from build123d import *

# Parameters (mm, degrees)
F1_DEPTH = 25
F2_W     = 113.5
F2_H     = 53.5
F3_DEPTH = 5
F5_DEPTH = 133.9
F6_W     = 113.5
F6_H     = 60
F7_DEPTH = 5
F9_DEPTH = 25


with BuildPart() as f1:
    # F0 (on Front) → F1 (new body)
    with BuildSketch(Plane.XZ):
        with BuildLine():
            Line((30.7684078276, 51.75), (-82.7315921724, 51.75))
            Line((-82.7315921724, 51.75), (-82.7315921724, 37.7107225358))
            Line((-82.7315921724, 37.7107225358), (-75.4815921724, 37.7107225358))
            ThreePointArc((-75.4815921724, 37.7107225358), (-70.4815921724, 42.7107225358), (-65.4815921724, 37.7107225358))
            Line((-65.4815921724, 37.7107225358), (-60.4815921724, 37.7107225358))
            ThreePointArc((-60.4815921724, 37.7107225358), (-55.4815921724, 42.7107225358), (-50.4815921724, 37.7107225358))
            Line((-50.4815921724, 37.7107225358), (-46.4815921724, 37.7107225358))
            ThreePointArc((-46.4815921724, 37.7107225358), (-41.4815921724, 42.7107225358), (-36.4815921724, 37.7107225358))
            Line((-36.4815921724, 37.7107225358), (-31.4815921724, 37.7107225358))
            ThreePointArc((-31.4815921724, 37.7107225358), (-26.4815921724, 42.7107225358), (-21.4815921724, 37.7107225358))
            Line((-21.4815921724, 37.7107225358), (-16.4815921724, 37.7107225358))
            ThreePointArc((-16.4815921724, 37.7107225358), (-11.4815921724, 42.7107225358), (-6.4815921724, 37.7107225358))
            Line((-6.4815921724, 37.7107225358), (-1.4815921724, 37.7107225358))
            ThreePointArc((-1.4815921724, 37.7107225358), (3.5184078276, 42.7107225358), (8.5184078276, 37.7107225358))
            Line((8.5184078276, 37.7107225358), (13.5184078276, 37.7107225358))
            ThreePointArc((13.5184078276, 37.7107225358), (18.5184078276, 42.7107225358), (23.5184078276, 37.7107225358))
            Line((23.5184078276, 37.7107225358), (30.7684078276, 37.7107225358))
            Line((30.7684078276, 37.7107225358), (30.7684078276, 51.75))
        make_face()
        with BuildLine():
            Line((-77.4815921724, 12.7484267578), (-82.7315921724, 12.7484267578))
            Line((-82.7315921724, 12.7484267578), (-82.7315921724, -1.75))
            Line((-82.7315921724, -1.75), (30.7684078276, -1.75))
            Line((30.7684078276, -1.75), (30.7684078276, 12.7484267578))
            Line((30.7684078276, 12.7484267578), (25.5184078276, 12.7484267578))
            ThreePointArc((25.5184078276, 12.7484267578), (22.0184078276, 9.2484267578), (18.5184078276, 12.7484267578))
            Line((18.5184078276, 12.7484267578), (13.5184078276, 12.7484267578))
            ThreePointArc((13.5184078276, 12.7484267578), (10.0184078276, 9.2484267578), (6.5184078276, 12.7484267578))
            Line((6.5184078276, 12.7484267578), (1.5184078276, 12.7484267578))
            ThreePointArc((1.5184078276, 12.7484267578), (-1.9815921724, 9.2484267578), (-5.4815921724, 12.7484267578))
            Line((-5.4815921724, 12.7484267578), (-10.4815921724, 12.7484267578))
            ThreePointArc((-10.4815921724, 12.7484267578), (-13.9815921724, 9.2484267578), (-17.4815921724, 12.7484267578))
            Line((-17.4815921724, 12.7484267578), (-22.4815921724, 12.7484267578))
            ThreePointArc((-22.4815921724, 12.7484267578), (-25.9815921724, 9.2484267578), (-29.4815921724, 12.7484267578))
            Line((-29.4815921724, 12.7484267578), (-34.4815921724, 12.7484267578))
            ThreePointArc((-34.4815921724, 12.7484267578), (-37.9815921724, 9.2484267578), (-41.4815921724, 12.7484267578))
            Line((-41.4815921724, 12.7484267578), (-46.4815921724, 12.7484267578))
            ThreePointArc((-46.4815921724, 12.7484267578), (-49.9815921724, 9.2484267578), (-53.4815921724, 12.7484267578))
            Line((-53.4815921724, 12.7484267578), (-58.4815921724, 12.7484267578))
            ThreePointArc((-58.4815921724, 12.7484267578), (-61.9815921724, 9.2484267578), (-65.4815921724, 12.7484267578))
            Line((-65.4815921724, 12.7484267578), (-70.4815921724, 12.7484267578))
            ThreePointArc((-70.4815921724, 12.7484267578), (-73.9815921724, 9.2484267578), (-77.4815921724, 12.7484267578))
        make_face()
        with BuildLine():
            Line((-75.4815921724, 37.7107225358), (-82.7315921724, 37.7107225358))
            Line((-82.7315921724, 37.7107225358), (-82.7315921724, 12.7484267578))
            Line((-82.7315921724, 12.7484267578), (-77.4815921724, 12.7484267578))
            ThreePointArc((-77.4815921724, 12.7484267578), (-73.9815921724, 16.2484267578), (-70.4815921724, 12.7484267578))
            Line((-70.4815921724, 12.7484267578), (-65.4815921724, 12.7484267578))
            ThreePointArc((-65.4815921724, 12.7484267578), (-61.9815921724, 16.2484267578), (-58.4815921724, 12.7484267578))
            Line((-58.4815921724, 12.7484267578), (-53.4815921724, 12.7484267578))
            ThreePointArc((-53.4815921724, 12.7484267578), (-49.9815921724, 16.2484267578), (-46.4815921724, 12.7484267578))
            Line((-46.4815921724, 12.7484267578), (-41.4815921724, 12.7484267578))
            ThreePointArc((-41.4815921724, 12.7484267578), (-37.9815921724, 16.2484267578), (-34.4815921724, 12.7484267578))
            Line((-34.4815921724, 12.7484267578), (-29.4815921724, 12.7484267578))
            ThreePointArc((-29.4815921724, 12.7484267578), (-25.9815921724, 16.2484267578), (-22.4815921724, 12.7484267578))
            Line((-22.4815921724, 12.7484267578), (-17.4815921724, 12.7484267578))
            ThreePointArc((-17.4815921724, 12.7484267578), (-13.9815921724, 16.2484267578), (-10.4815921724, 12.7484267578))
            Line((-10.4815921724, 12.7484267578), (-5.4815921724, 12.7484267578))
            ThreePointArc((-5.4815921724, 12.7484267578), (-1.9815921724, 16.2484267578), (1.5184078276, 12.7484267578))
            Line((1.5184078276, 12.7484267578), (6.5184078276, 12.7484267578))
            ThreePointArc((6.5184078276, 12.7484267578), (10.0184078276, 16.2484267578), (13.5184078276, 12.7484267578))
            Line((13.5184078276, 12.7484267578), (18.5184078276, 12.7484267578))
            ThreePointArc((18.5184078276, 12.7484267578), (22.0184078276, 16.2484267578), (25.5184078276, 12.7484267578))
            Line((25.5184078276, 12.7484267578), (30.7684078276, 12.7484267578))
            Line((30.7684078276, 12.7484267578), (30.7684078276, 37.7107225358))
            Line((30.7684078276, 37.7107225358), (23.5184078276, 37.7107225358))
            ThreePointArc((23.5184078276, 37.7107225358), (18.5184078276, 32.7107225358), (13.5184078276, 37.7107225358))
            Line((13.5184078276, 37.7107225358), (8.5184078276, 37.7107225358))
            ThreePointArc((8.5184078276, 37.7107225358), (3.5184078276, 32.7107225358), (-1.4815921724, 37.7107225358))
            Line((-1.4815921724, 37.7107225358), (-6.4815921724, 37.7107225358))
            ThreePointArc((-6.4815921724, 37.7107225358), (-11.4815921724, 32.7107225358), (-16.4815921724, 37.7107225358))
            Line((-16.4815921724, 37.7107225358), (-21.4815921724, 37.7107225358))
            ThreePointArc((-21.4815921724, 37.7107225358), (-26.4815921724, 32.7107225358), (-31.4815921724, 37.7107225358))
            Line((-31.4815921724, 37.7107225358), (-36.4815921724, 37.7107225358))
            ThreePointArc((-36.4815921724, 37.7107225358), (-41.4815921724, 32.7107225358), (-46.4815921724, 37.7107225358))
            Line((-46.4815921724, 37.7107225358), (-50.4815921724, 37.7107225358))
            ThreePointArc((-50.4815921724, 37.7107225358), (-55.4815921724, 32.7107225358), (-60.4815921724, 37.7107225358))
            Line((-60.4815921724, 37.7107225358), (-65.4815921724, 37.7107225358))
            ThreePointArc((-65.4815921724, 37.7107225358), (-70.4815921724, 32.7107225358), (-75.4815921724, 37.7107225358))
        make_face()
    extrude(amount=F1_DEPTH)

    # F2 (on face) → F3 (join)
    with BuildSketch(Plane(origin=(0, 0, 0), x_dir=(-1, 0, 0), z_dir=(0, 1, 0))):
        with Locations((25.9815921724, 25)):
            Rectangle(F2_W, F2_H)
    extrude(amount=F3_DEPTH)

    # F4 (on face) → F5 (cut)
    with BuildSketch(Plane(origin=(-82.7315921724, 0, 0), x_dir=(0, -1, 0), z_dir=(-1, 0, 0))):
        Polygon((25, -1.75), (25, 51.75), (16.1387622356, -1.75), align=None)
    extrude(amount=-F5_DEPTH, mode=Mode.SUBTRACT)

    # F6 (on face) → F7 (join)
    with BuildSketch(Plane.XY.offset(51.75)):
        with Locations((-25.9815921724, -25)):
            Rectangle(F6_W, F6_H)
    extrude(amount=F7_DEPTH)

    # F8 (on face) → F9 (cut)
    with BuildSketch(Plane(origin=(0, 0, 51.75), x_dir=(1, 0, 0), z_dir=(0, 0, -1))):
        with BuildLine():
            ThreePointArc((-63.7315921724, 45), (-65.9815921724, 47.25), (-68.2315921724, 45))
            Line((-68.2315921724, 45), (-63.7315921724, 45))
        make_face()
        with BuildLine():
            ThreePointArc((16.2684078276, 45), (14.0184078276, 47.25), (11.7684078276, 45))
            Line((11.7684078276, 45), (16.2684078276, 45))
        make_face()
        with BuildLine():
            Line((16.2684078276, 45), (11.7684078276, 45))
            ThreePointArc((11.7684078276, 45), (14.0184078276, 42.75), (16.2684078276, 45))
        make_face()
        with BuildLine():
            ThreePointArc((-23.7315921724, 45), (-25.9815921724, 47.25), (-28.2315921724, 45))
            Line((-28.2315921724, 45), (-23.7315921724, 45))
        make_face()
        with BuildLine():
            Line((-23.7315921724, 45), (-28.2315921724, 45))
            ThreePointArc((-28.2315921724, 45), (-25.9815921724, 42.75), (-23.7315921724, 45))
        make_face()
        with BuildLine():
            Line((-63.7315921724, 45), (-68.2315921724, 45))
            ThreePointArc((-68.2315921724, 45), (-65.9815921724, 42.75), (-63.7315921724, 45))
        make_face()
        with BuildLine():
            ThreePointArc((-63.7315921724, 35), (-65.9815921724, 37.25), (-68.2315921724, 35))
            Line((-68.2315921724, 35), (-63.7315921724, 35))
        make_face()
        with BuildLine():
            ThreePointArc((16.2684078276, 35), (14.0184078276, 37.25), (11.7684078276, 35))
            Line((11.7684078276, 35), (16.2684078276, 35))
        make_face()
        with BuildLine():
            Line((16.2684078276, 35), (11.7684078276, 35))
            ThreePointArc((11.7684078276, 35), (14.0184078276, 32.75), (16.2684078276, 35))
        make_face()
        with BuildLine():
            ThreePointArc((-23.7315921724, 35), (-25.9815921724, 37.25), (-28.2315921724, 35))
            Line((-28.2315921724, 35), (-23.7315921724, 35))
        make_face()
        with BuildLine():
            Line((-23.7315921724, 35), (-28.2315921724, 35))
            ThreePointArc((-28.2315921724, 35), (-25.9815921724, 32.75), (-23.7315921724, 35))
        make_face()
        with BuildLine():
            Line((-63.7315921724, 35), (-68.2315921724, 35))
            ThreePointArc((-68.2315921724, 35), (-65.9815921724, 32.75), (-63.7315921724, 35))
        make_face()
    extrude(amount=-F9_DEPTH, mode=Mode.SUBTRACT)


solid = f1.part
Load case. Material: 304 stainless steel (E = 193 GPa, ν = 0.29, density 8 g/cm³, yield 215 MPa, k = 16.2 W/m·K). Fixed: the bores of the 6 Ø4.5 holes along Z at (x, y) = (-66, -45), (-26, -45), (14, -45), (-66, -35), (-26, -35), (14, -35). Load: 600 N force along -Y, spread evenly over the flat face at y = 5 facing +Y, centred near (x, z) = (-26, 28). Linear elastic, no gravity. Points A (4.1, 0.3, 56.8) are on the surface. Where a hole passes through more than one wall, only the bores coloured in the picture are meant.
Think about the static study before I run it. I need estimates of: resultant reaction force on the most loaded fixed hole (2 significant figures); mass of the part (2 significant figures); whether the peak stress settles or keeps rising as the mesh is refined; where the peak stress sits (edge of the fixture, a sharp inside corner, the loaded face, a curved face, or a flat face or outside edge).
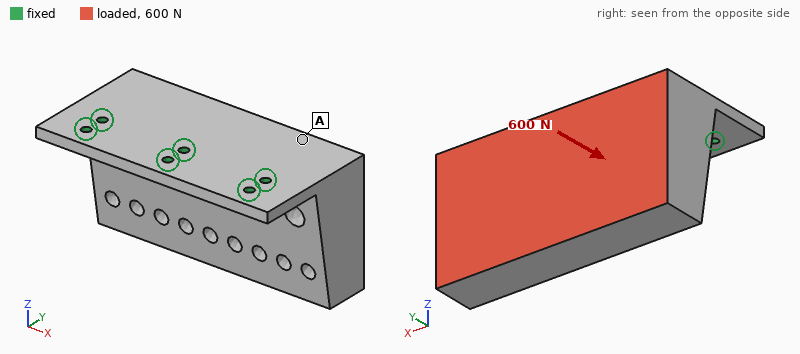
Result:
260 N
1.4 kg
keeps rising
edge of the fixture
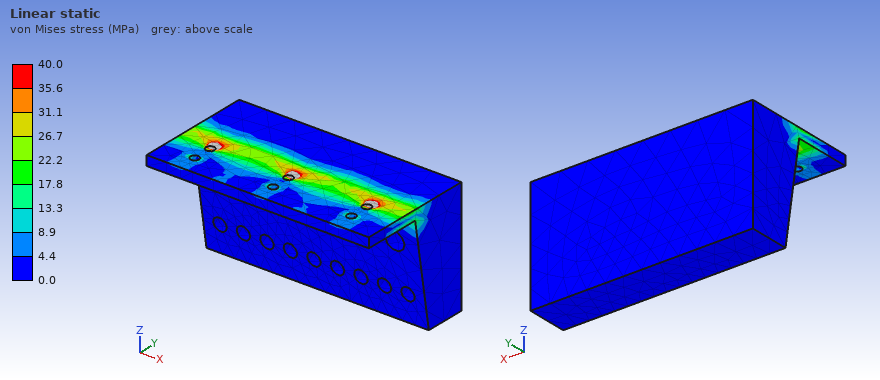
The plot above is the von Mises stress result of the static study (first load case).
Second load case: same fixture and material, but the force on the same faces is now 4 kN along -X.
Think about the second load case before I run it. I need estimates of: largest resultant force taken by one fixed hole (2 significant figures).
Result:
2.3 kN
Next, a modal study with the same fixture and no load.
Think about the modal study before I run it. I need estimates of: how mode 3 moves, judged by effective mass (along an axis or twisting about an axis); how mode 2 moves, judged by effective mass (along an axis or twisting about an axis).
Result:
along Z
along X
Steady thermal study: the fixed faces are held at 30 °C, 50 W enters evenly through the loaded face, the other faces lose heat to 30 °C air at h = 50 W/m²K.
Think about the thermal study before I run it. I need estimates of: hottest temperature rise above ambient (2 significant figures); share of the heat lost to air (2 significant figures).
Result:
42 K
79 %
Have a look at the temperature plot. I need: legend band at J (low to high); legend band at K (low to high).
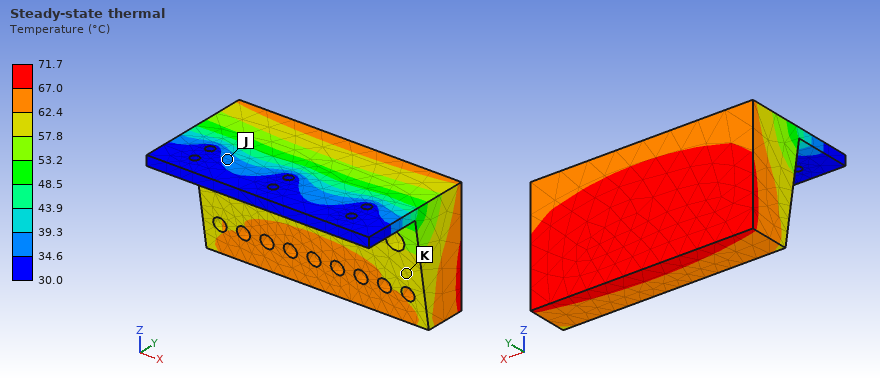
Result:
34.6 to 39.3 °C
57.8 to 62.4 °C
